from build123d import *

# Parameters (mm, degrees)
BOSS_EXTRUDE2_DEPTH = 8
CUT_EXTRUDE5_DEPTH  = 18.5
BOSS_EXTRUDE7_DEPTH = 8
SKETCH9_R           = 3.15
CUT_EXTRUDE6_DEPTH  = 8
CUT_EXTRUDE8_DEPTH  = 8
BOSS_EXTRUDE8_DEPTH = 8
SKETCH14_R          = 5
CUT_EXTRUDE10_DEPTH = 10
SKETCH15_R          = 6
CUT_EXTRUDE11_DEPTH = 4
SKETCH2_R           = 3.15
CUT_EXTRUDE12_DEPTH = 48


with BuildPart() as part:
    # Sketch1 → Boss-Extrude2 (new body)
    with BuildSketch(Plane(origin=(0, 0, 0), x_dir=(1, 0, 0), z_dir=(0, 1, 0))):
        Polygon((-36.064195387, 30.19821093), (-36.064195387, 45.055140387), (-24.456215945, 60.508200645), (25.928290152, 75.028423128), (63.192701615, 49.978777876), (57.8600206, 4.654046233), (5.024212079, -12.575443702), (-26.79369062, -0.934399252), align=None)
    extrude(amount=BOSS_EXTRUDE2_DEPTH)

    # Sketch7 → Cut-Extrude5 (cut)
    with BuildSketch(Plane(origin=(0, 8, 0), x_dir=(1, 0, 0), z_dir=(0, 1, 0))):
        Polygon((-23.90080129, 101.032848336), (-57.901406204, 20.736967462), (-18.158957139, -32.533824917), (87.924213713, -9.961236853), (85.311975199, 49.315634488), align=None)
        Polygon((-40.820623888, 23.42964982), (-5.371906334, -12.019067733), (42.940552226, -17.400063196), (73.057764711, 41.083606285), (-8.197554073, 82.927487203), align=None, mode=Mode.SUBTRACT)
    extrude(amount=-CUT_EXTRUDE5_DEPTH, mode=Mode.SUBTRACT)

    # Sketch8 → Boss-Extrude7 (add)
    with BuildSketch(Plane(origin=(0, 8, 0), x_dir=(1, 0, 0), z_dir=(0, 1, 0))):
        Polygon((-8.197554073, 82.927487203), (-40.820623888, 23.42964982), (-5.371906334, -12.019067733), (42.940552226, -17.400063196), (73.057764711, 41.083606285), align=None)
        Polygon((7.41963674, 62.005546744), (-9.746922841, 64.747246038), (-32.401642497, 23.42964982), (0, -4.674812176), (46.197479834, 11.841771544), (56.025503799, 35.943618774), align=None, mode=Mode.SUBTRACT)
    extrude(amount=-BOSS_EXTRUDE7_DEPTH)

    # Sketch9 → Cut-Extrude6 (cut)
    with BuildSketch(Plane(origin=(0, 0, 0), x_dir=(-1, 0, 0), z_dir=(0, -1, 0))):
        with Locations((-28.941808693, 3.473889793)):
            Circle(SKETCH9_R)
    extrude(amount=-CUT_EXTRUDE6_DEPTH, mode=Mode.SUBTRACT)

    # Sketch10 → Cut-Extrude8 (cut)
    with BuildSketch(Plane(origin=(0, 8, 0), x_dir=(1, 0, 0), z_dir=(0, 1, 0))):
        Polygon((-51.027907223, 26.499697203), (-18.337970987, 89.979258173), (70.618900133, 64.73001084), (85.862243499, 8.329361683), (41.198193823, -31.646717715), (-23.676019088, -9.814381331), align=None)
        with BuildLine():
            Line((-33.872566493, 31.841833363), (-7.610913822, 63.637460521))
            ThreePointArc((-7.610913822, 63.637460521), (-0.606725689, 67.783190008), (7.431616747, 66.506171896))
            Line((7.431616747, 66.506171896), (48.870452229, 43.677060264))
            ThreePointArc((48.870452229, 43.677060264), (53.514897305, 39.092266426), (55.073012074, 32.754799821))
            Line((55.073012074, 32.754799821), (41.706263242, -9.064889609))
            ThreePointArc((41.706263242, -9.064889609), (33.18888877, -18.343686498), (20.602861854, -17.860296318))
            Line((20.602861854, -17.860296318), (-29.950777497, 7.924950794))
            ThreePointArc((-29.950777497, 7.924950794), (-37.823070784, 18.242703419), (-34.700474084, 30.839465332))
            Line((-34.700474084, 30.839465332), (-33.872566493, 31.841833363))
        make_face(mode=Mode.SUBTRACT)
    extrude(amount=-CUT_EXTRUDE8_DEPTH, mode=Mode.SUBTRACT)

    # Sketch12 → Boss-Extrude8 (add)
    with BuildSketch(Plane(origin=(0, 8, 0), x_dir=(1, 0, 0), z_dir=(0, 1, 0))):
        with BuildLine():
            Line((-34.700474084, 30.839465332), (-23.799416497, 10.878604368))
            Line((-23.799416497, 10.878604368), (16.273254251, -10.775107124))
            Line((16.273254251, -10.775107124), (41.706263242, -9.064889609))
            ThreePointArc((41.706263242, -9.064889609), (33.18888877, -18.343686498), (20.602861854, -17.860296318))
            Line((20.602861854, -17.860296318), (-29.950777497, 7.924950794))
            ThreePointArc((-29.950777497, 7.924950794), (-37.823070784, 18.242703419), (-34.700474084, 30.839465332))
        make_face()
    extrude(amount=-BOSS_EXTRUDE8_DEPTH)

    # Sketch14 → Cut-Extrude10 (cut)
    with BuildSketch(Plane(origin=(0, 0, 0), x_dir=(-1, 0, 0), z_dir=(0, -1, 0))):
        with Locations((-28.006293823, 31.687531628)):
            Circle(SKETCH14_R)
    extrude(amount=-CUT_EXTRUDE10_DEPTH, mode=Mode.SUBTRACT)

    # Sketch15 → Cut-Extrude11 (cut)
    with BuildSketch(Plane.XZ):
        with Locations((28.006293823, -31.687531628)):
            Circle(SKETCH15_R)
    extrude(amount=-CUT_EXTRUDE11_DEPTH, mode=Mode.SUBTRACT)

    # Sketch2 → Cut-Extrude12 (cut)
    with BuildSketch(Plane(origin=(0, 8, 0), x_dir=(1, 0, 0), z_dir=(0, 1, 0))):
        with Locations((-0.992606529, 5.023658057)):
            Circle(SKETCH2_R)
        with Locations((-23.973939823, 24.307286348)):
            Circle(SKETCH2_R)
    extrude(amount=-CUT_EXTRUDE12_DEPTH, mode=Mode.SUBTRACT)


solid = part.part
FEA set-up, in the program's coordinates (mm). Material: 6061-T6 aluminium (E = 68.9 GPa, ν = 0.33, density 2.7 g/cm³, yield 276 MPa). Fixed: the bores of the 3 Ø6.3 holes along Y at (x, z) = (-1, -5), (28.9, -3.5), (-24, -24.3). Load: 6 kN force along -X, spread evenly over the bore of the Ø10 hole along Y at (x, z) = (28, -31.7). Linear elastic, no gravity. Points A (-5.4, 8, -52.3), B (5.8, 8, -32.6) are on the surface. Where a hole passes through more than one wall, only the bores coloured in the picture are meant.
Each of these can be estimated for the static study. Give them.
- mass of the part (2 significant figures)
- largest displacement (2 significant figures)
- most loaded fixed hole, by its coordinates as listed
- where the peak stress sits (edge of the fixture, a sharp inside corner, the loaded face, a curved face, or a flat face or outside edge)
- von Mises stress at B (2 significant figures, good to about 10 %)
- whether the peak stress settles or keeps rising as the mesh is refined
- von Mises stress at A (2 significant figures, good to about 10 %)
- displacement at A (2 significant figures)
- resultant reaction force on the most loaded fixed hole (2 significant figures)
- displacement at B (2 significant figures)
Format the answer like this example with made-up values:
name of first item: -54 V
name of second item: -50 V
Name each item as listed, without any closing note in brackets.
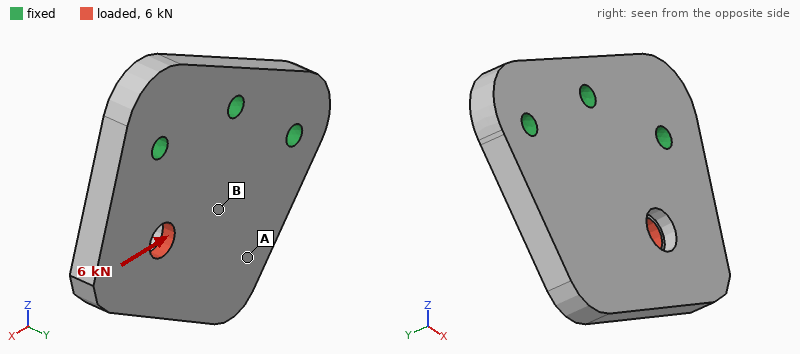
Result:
mass of the part: 110 g
largest displacement: 40 µm
most loaded fixed hole, by its coordinates as listed: (-24, -24.3)
where the peak stress sits: a sharp inside corner
von Mises stress at B: 24 MPa
whether the peak stress settles or keeps rising as the mesh is refined: keeps rising
von Mises stress at A: 9.4 MPa
displacement at A: 12 µm
resultant reaction force on the most loaded fixed hole: 3.3 kN
displacement at B: 9.0 µm
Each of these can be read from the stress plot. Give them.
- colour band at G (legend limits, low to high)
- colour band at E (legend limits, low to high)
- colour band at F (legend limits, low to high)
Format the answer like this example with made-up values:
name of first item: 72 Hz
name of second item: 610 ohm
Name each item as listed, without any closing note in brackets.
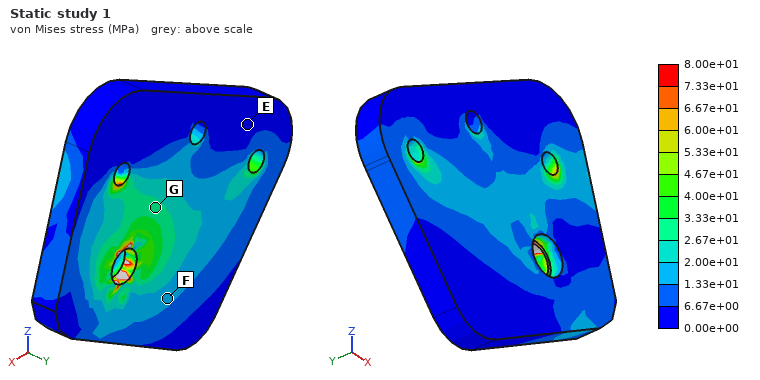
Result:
colour band at G: 2.67e+01 to 3.33e+01 MPa
colour band at E: 0.00e+00 to 6.67e+00 MPa
colour band at F: 1.33e+01 to 2.00e+01 MPa
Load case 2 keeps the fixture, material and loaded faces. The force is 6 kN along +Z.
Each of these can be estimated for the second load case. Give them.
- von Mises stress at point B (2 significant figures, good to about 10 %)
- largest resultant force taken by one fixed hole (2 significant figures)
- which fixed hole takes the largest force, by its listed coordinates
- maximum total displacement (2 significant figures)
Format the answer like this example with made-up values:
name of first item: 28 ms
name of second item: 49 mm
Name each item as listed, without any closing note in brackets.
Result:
von Mises stress at point B: 15 MPa
largest resultant force taken by one fixed hole: 5.0 kN
which fixed hole takes the largest force, by its listed coordinates: (28.9, -3.5)
maximum total displacement: 56 µm
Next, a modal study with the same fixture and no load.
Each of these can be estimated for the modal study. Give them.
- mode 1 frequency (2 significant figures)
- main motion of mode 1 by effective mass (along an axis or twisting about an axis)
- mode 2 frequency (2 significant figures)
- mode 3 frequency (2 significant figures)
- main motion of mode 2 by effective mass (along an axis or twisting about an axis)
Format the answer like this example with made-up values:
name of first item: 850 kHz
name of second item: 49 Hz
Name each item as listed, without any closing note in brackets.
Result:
mode 1 frequency: 2800 Hz
main motion of mode 1 by effective mass: along Y
mode 2 frequency: 5500 Hz
mode 3 frequency: 11 kHz
main motion of mode 2 by effective mass: twisting about Z
